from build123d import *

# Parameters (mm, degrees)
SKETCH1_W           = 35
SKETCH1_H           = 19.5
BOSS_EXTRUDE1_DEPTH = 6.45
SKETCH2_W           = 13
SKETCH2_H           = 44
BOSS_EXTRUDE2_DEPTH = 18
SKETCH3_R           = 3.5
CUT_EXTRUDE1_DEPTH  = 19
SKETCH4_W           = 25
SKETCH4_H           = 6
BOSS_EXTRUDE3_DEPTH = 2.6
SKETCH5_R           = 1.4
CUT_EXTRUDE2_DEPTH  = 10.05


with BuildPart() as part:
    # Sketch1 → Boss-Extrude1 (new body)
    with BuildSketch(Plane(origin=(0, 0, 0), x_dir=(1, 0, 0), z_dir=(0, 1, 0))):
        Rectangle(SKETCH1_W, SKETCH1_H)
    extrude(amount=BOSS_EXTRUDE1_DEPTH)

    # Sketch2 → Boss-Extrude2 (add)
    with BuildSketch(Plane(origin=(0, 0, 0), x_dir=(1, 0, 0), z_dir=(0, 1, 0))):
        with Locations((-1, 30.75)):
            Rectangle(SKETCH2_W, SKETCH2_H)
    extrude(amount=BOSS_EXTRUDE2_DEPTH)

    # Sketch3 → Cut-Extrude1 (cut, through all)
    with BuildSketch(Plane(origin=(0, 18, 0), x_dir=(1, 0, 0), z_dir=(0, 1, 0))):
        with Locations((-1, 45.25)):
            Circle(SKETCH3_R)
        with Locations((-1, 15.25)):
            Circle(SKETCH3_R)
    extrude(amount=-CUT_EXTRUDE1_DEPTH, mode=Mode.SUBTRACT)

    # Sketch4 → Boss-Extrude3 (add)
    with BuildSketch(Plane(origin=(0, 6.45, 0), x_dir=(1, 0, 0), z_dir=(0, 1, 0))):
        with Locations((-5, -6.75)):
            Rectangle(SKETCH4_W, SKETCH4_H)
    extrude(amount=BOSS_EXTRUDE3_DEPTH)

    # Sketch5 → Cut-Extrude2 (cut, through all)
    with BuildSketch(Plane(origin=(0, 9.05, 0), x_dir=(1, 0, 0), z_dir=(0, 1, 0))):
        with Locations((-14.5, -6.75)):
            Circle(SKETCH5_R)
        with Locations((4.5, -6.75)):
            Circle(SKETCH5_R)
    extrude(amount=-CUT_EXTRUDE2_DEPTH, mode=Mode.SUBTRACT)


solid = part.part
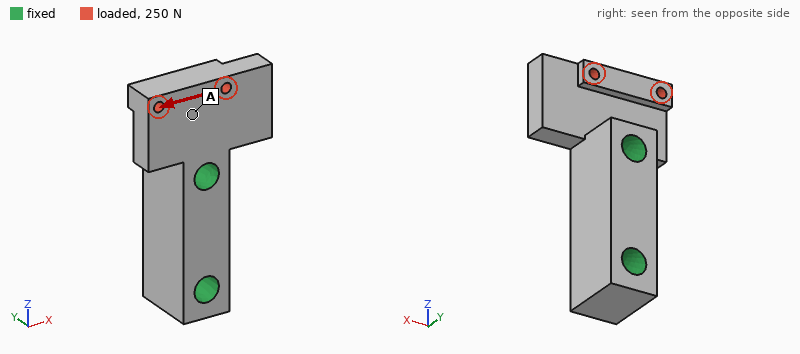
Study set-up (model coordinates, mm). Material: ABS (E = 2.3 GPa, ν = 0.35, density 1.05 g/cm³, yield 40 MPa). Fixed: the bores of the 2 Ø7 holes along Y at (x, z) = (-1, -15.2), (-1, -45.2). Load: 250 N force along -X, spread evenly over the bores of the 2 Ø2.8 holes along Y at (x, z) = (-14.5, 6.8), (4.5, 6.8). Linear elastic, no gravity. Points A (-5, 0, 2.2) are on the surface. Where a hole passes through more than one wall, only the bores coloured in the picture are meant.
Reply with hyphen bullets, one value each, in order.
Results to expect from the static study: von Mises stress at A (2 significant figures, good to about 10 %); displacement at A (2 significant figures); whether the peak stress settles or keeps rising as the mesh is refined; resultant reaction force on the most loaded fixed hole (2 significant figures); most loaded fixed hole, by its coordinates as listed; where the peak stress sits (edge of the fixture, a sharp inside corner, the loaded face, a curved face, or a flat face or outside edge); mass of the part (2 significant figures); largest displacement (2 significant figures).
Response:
- 3.0 MPa
- 0.21 mm
- keeps rising
- 270 N
- (-1, -15.2)
- a sharp inside corner
- 14 g
- 0.45 mm
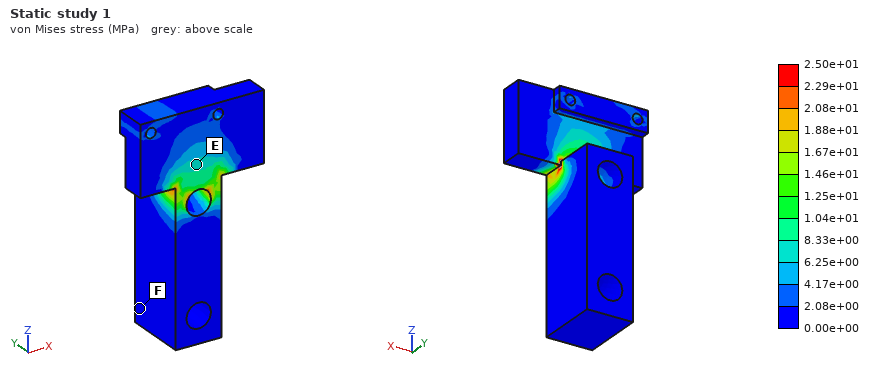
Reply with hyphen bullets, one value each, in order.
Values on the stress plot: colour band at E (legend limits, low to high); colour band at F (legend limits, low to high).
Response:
- 6.25e+00 to 8.33e+00 MPa
- 0.00e+00 to 2.08e+00 MPa
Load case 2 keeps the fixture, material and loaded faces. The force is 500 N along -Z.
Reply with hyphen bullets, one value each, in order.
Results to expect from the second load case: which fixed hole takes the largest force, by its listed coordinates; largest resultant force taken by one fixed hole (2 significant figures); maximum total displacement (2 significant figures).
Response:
- (-1, -15.2)
- 490 N
- 0.30 mm
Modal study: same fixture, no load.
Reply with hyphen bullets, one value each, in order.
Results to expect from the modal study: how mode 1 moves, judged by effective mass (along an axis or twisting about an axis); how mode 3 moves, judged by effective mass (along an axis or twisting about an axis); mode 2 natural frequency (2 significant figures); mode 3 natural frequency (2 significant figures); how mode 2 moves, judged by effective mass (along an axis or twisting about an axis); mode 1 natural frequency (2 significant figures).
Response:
- along Y
- twisting about Z
- 2400 Hz
- 2700 Hz
- along X
- 2100 Hz
